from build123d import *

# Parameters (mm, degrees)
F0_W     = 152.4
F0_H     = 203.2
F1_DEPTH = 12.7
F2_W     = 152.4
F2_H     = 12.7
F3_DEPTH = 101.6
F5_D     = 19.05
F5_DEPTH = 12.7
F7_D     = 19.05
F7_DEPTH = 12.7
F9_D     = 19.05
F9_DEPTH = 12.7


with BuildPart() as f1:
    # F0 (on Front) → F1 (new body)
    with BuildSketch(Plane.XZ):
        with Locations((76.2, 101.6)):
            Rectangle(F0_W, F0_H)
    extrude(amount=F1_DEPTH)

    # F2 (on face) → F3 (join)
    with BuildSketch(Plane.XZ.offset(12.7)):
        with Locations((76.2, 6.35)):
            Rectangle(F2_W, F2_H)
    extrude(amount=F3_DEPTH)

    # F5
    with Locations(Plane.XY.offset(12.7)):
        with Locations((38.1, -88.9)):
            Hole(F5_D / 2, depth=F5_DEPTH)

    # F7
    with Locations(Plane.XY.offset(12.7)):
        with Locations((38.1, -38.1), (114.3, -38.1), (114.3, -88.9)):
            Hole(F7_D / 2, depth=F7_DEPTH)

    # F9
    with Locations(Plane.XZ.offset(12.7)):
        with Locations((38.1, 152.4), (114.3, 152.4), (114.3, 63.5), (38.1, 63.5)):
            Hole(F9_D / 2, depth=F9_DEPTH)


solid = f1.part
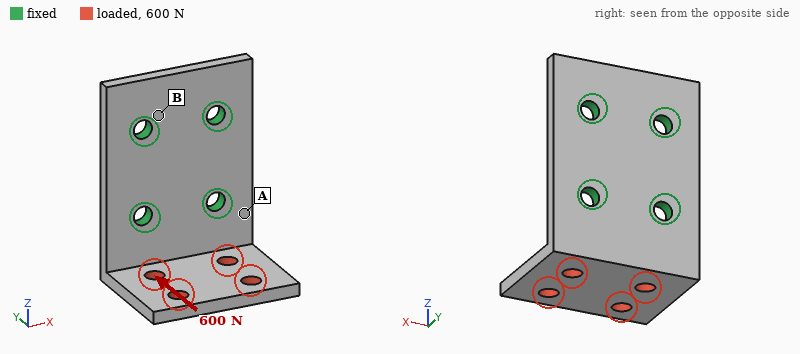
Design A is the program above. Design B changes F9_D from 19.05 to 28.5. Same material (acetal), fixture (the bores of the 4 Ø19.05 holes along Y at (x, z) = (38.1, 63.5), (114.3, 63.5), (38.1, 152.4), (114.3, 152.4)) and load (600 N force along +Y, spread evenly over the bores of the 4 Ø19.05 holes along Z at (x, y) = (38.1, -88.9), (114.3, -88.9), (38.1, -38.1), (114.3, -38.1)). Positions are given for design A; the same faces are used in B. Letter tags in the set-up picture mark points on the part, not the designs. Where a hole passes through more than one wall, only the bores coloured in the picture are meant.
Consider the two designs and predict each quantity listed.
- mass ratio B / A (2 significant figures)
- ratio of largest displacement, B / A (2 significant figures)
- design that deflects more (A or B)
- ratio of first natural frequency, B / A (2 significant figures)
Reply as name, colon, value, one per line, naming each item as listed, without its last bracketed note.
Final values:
mass ratio B / A: 0.97
ratio of largest displacement, B / A: 0.79
design that deflects more: A
ratio of first natural frequency, B / A: 1.1
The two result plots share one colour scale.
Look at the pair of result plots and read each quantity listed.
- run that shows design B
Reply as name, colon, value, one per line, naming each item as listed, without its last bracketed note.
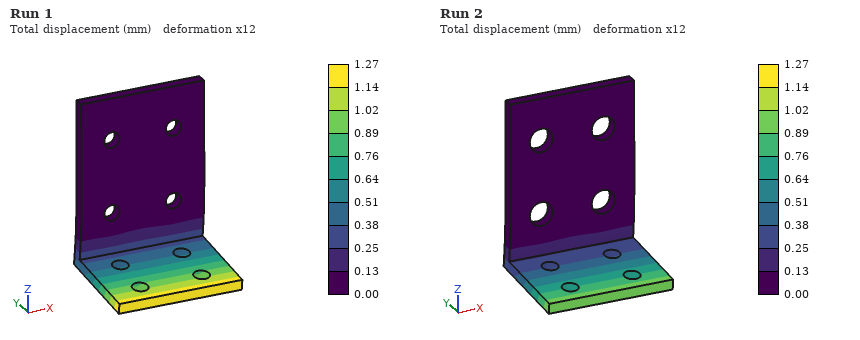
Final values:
run that shows design B: Run 2
